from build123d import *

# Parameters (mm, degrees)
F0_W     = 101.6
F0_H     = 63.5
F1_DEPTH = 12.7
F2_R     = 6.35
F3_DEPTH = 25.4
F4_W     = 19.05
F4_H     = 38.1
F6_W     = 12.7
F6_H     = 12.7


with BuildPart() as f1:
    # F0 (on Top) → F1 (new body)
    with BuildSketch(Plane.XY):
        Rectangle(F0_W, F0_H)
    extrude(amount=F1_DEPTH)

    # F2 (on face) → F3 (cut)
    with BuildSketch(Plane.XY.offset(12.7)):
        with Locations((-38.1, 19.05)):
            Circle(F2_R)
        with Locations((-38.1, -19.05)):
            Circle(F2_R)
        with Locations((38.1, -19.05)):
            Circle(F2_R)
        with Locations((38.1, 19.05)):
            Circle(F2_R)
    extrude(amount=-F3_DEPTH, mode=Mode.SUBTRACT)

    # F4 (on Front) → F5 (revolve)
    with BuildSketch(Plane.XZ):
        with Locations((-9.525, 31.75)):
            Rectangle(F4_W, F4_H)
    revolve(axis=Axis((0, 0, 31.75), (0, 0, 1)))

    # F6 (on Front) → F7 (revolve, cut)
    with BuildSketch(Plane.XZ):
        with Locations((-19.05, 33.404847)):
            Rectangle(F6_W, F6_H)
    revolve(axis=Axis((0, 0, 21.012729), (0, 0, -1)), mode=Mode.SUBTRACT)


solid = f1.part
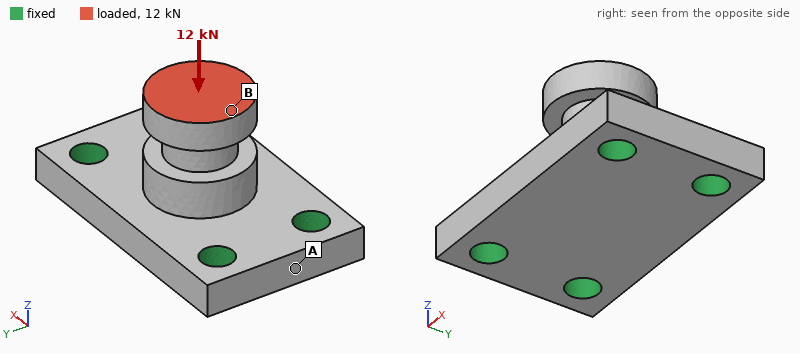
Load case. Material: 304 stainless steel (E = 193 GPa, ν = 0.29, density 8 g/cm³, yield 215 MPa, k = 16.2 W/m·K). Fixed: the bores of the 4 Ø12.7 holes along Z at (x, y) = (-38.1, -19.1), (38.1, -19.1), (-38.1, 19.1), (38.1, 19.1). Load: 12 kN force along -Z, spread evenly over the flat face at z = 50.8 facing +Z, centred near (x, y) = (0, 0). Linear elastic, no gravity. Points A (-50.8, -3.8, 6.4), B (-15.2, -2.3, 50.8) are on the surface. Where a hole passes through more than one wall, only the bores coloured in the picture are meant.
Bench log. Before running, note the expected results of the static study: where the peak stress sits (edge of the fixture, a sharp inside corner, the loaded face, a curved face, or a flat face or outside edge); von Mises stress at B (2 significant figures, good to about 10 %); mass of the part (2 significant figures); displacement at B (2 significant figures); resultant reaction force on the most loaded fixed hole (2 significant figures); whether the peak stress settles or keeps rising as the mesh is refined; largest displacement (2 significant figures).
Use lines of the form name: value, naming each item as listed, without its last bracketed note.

where the peak stress sits: edge of the fixture
von Mises stress at B: 16 MPa
mass of the part: 890 g
displacement at B: 12 µm
resultant reaction force on the most loaded fixed hole: 3.1 kN
whether the peak stress settles or keeps rising as the mesh is refined: keeps rising
largest displacement: 12 µm
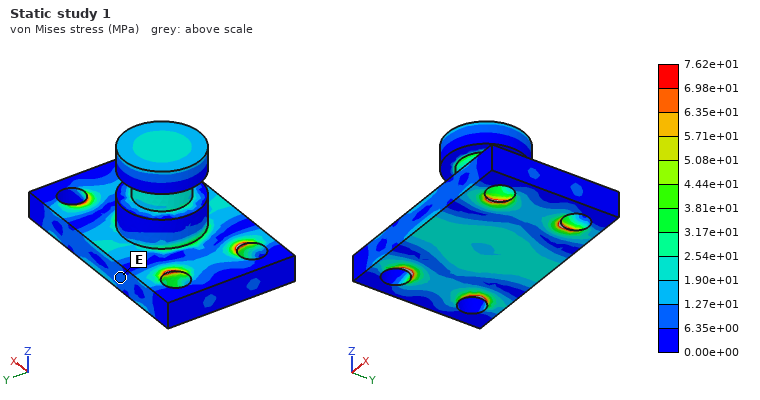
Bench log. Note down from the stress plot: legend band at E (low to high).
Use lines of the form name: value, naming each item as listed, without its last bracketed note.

legend band at E: 6.35e+00 to 1.27e+01 MPa
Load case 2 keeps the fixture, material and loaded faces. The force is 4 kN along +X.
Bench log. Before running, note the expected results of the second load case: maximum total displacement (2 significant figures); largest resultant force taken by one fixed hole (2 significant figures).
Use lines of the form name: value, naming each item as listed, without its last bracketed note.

maximum total displacement: 24 µm
largest resultant force taken by one fixed hole: 2.0 kN
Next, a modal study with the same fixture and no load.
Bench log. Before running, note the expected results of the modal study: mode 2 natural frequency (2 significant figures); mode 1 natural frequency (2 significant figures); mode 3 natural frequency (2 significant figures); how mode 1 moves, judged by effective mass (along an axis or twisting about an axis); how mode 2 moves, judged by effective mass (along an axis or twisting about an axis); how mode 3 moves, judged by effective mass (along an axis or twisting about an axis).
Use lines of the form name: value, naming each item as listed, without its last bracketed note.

mode 2 natural frequency: 7200 Hz
mode 1 natural frequency: 5600 Hz
mode 3 natural frequency: 8500 Hz
how mode 1 moves, judged by effective mass: along Y
how mode 2 moves, judged by effective mass: along X
how mode 3 moves, judged by effective mass: along Z
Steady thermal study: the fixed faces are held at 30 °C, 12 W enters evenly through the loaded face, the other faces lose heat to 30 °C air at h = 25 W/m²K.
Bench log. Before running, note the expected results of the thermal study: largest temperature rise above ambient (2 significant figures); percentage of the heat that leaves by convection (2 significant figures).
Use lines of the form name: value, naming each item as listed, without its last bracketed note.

largest temperature rise above ambient: 43 K
percentage of the heat that leaves by convection: 37 %
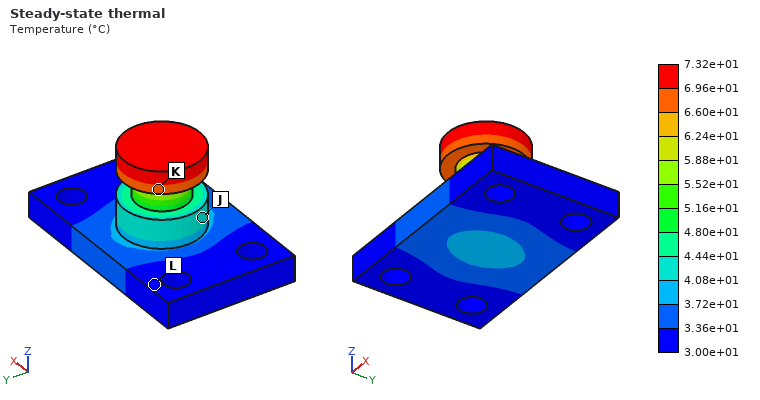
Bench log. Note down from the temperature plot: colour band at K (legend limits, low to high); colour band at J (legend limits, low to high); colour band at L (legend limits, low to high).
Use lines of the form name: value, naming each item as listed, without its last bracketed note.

colour band at K: 6.60e+01 to 6.96e+01 °C
colour band at J: 4.08e+01 to 4.44e+01 °C
colour band at L: 3.00e+01 to 3.36e+01 °C
